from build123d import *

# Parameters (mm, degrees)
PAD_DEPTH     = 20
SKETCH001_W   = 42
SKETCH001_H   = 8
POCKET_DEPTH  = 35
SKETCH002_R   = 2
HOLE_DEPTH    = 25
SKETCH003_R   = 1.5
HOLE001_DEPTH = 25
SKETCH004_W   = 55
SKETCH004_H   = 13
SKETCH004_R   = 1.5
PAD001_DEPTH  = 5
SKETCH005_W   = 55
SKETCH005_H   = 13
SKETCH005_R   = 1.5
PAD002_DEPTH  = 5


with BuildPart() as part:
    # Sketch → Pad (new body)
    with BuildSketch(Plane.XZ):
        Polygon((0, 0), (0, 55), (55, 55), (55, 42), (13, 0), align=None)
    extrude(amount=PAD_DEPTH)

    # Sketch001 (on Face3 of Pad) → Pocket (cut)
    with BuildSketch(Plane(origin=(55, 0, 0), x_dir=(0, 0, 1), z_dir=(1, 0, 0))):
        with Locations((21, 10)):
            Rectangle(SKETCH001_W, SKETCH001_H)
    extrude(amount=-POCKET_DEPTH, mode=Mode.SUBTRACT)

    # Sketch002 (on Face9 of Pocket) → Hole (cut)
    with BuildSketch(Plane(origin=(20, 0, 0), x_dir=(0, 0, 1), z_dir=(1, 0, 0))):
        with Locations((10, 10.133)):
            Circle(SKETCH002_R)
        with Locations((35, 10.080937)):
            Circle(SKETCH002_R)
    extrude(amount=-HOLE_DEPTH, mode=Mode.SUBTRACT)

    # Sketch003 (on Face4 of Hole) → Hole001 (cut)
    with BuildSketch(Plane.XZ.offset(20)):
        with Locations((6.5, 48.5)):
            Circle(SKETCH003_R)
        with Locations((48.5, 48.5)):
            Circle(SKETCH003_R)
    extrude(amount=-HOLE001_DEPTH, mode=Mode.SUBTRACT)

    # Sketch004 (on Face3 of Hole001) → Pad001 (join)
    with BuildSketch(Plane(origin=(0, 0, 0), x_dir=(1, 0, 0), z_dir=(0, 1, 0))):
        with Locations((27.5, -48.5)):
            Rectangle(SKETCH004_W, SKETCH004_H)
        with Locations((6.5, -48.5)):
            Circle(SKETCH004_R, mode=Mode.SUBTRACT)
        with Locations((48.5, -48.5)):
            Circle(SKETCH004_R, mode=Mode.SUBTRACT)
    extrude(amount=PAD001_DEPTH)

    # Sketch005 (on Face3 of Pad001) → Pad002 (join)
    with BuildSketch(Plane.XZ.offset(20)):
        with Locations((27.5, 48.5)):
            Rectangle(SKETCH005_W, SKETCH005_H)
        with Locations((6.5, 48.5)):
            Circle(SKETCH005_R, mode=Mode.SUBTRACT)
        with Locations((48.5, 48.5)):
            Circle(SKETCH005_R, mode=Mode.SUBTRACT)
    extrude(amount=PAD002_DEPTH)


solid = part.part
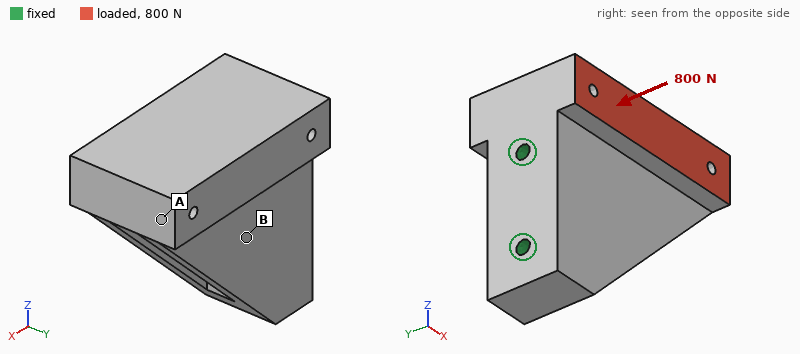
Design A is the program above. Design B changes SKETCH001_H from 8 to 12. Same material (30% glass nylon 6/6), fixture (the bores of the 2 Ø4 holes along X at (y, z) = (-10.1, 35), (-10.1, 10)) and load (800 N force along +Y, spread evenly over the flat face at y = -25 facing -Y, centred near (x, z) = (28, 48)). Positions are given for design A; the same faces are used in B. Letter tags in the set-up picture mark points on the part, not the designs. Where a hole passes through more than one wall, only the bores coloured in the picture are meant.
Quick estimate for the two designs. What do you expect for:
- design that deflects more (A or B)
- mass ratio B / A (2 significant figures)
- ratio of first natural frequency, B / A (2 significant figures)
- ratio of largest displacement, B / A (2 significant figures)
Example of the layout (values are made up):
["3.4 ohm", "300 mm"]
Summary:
["B", "0.94", "0.96", "1.1"]
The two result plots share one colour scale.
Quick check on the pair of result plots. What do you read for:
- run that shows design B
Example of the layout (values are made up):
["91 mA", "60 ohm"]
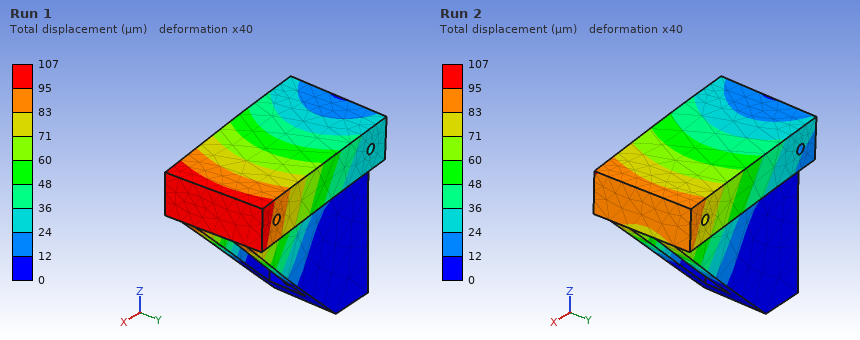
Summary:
["Run 1"]
